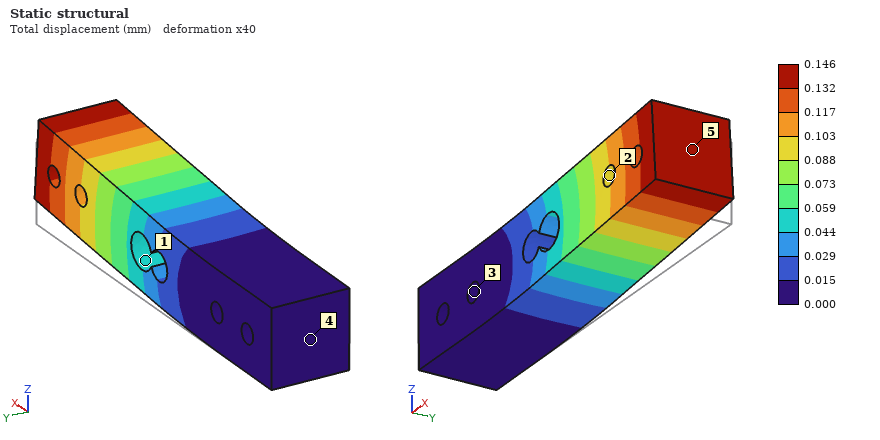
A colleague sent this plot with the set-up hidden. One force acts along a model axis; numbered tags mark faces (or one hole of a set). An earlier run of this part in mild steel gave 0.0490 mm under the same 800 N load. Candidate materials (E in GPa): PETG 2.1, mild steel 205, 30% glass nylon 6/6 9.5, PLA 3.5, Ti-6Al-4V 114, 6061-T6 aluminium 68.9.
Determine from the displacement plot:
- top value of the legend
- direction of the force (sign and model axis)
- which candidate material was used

0.146 mm
+Z
6061-T6 aluminium
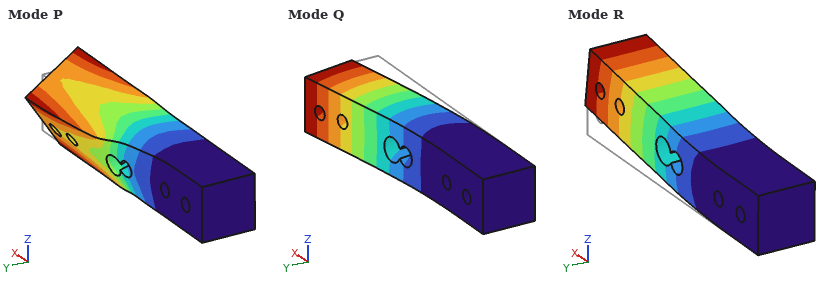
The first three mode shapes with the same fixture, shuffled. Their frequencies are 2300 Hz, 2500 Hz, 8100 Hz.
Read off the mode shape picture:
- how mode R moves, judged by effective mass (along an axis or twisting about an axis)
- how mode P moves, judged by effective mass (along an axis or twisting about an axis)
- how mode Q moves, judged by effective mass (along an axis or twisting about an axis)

along Z
twisting about X
along Y
